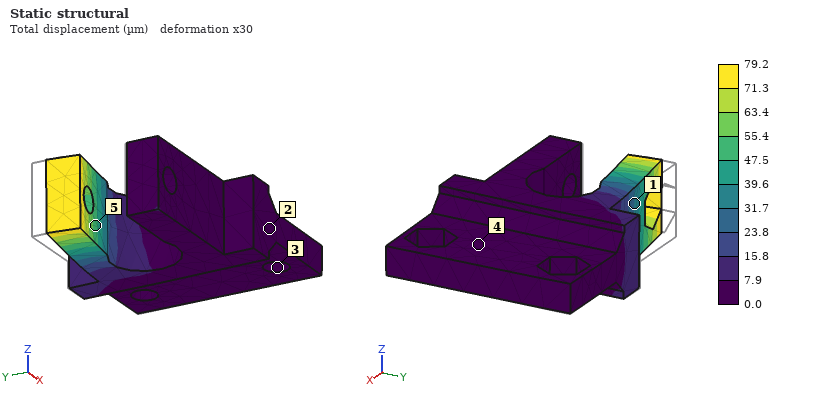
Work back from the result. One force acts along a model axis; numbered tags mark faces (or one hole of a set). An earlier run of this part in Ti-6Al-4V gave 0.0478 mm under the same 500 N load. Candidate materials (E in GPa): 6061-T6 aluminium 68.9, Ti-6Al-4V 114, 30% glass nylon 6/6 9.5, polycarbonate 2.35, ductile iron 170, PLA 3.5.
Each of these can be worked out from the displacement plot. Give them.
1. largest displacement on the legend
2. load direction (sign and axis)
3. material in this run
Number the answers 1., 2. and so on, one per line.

1. 79.2 µm
2. -Y
3. 6061-T6 aluminium
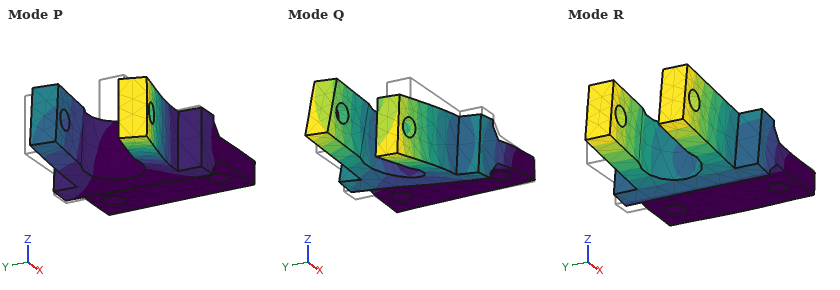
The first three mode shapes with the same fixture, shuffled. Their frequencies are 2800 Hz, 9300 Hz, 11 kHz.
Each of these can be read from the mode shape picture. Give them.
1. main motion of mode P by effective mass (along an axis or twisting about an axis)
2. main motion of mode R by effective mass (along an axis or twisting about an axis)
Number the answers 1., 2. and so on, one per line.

1. along Y
2. along Z
